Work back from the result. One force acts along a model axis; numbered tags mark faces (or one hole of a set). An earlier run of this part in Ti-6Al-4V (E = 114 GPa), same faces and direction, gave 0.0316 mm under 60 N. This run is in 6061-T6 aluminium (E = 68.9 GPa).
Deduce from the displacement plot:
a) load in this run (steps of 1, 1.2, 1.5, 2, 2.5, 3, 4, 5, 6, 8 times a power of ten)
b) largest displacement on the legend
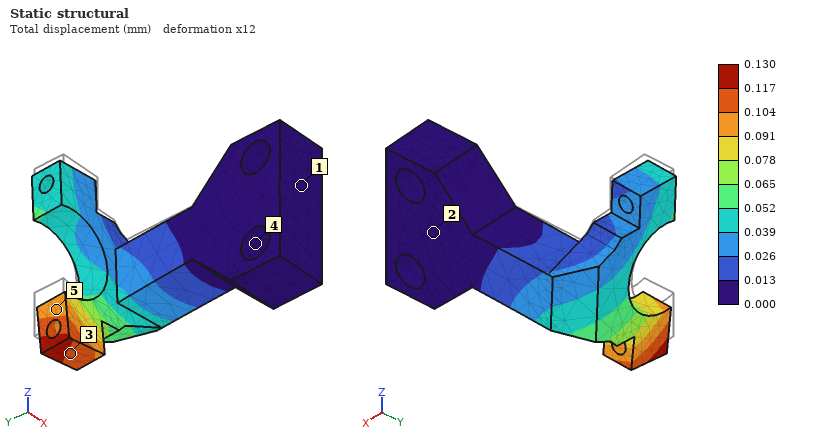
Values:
150 N
0.130 mm
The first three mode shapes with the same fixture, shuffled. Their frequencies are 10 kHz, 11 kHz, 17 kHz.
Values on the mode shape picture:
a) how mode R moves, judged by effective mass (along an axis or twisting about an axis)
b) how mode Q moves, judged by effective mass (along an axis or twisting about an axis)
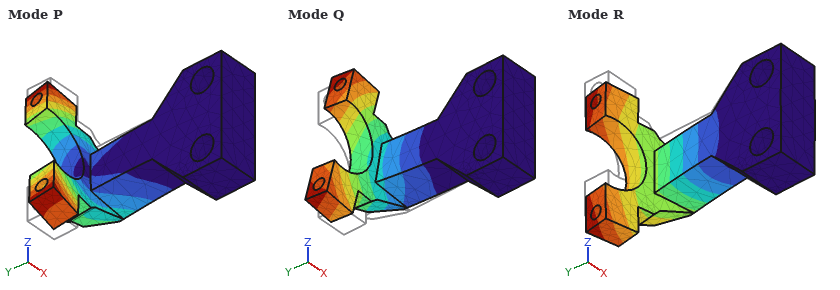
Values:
along X
along Z
